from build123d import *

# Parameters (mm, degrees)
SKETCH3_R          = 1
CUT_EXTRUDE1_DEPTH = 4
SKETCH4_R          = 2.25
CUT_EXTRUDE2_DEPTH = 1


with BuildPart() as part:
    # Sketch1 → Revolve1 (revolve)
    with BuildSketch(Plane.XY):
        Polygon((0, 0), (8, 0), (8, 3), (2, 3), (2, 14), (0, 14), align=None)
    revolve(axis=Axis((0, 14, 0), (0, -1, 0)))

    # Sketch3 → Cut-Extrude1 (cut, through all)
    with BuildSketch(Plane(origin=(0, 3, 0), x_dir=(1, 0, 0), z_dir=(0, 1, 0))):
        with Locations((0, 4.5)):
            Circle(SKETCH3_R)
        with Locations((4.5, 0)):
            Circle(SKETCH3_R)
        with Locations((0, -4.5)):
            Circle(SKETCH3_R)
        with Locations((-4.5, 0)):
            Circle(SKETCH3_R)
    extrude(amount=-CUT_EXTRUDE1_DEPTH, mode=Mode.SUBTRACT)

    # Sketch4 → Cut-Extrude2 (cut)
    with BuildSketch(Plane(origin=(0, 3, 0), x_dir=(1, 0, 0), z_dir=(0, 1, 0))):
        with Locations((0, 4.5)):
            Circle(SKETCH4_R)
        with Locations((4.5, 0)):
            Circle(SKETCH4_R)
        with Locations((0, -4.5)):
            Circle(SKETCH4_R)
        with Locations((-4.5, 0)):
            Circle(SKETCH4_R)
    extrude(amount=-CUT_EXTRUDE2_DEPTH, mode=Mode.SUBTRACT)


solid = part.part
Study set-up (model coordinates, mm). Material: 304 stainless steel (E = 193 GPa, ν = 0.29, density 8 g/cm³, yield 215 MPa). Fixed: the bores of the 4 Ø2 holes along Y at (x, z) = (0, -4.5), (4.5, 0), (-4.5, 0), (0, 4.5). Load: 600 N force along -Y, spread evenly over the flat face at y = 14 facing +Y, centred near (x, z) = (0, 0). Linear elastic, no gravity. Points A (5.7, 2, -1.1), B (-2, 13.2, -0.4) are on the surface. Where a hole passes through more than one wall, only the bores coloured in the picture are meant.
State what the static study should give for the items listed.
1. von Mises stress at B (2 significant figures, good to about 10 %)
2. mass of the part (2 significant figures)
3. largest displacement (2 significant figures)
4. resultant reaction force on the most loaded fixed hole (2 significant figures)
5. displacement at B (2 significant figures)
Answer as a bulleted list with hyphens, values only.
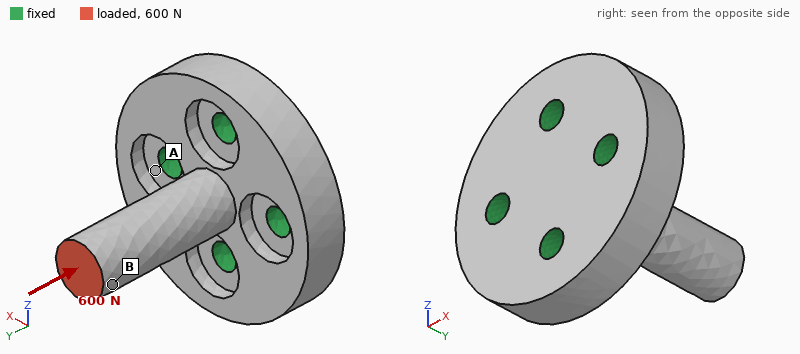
- 48 MPa
- 5.2 g
- 3.7 µm
- 160 N
- 3.5 µm
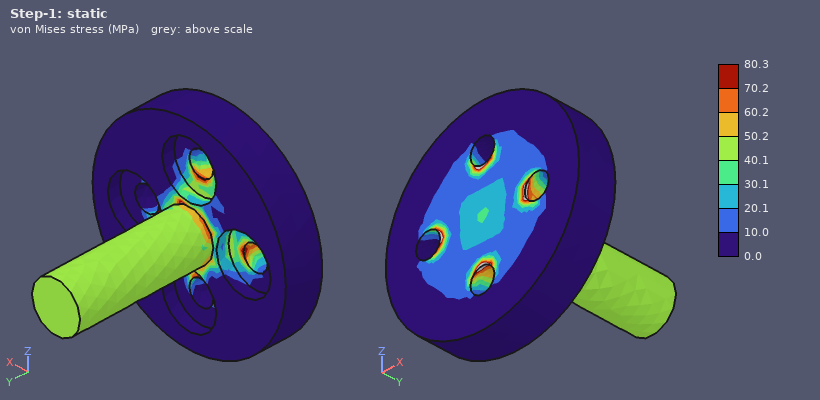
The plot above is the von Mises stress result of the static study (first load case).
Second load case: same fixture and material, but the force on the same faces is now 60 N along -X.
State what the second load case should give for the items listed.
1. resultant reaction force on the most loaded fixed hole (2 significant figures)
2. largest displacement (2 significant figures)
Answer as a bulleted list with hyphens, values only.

- 95 N
- 16 µm
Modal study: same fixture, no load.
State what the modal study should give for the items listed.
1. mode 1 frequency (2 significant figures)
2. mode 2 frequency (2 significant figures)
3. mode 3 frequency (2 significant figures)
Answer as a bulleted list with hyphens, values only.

- 18 kHz
- 18 kHz
- 65 kHz
